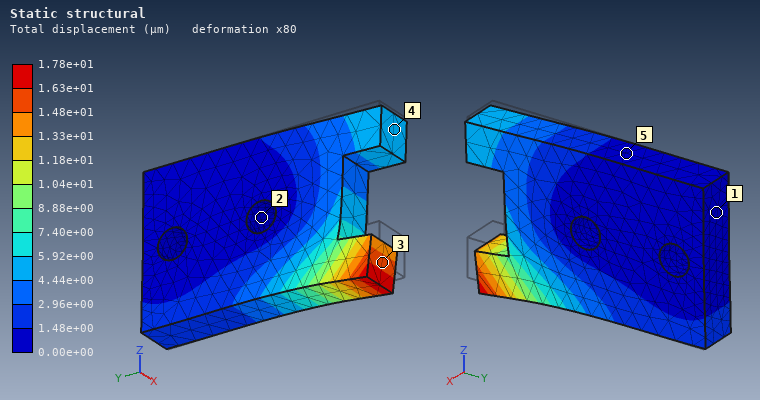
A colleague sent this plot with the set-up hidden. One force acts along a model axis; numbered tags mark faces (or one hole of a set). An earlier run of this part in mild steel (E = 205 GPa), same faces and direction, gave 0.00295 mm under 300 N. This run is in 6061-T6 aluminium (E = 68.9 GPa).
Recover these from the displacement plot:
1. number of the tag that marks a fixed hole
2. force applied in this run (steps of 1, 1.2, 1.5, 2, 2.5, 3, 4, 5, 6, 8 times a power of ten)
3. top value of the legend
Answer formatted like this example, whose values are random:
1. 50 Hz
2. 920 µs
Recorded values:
1. 2
2. 600 N
3. 1.78e+01 µm
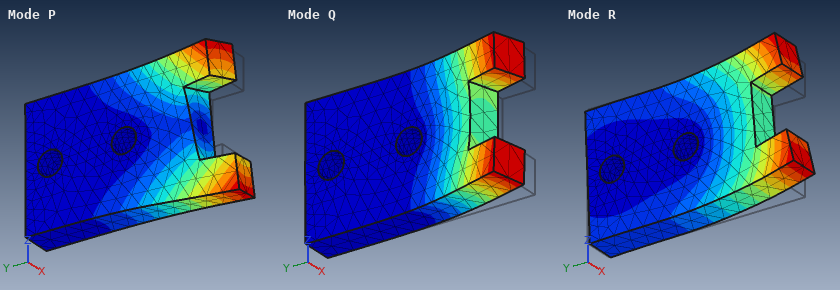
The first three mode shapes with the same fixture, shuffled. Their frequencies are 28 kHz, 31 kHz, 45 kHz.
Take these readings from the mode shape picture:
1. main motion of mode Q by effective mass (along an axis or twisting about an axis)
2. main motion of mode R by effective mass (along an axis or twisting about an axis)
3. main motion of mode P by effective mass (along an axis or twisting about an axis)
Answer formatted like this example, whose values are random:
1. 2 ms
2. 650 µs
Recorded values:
1. along X
2. along Z
3. twisting about Y
